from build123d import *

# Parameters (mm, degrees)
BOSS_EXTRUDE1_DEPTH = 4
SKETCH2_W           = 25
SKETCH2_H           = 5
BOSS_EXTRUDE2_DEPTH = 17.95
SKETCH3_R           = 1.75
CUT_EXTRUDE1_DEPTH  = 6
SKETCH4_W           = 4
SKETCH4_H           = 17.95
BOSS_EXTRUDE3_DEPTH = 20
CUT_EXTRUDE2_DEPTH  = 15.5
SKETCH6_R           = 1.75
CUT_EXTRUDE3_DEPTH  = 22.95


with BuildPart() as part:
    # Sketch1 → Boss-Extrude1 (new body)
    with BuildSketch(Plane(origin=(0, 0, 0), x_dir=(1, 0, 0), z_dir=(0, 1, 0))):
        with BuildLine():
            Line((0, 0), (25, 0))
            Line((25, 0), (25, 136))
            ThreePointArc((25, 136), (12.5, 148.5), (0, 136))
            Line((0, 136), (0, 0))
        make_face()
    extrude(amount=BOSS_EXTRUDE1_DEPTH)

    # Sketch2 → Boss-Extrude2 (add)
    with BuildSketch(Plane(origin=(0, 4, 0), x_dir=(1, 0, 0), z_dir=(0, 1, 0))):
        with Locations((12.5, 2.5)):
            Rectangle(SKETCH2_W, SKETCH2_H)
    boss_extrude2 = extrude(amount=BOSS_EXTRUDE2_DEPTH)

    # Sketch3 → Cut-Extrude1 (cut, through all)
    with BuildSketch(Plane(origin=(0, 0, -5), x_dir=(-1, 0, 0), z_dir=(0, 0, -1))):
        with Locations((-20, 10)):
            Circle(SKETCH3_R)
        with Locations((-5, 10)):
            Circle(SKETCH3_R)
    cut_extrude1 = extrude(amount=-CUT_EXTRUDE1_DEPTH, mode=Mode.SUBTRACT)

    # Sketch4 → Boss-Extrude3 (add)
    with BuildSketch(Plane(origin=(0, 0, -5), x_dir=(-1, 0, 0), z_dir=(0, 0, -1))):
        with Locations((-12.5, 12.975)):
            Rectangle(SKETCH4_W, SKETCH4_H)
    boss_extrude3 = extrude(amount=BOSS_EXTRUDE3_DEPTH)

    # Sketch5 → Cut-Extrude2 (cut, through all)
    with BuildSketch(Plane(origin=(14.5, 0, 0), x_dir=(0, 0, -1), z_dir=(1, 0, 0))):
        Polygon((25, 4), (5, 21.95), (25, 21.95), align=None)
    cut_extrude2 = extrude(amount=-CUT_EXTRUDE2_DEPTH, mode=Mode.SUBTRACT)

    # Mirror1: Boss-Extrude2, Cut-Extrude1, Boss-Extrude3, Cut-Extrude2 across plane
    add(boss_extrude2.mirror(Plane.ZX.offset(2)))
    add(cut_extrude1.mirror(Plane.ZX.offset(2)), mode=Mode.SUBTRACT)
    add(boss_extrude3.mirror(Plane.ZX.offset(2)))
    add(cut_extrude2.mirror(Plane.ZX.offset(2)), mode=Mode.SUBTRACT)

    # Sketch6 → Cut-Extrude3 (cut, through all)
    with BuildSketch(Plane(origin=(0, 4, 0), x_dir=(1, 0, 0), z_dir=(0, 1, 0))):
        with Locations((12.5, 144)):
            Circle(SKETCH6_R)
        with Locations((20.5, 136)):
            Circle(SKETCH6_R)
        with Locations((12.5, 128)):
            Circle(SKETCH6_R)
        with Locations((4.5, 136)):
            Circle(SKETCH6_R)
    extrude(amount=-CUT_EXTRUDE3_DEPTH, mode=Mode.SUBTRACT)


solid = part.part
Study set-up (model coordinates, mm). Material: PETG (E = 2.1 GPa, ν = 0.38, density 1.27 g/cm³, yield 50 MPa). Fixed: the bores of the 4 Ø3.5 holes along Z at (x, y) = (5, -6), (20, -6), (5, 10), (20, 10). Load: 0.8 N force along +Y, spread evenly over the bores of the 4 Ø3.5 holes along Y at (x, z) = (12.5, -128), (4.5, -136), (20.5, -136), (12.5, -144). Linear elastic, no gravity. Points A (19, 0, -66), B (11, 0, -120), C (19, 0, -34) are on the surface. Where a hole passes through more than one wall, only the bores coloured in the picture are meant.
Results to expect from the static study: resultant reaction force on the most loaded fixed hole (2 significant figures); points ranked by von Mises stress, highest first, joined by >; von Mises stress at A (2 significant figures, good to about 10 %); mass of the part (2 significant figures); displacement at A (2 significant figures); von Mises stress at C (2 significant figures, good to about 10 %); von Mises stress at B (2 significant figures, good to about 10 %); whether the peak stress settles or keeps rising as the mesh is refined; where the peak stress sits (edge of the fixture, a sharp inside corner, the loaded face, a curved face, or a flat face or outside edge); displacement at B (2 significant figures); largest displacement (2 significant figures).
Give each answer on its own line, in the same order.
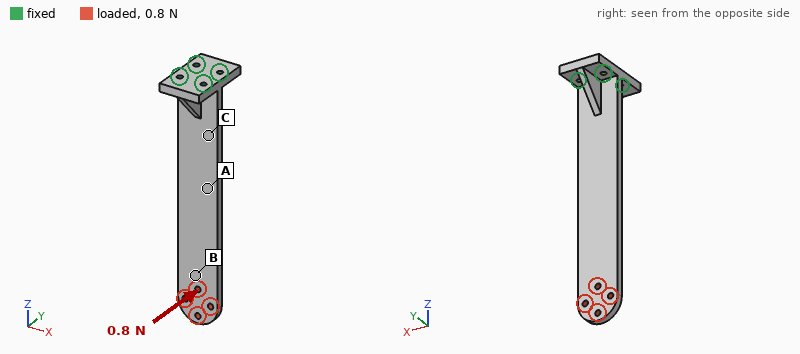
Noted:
2.5 N
C > A > B
0.84 MPa
26 g
0.30 mm
1.2 MPa
0.19 MPa
keeps rising
a sharp inside corner
1.2 mm
1.7 mm
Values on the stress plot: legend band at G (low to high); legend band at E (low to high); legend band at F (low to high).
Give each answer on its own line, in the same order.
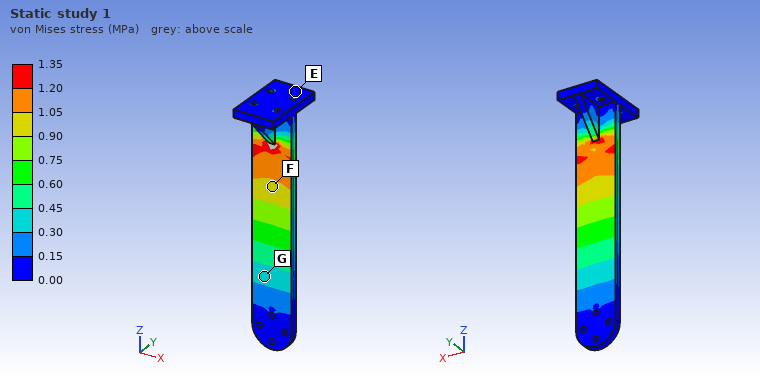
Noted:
0.30 to 0.45 MPa
0.00 to 0.15 MPa
0.90 to 1.05 MPa
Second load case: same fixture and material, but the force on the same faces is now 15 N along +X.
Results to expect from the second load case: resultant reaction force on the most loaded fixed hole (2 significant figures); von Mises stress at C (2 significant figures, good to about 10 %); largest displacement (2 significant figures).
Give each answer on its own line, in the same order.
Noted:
59 N
1.9 MPa
1.5 mm
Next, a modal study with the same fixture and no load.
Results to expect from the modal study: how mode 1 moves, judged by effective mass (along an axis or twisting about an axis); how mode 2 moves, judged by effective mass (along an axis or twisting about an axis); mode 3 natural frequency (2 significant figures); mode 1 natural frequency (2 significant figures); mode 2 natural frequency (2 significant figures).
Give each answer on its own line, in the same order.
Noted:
along Y
along X
330 Hz
54 Hz
230 Hz
